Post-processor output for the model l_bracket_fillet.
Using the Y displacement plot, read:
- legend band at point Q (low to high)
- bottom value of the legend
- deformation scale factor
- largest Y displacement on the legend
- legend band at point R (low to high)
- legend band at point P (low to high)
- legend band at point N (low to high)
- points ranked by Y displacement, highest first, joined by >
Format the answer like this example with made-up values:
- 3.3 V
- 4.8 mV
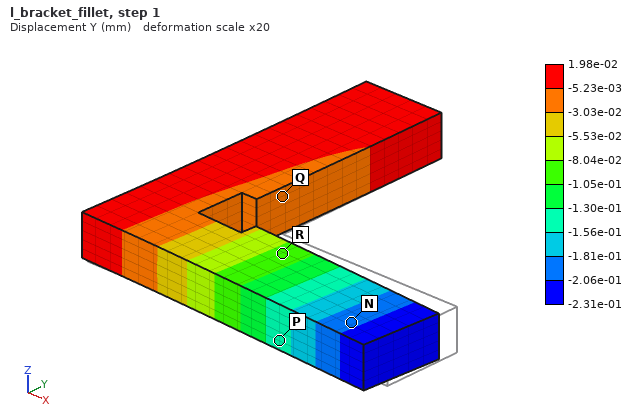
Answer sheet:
- -3.03e-02 to -5.23e-03 mm
- -2.31e-01 mm
- 20
- 1.98e-02 mm
- -1.05e-01 to -8.04e-02 mm
- -1.56e-01 to -1.30e-01 mm
- -2.06e-01 to -1.81e-01 mm
- Q > R > P > N
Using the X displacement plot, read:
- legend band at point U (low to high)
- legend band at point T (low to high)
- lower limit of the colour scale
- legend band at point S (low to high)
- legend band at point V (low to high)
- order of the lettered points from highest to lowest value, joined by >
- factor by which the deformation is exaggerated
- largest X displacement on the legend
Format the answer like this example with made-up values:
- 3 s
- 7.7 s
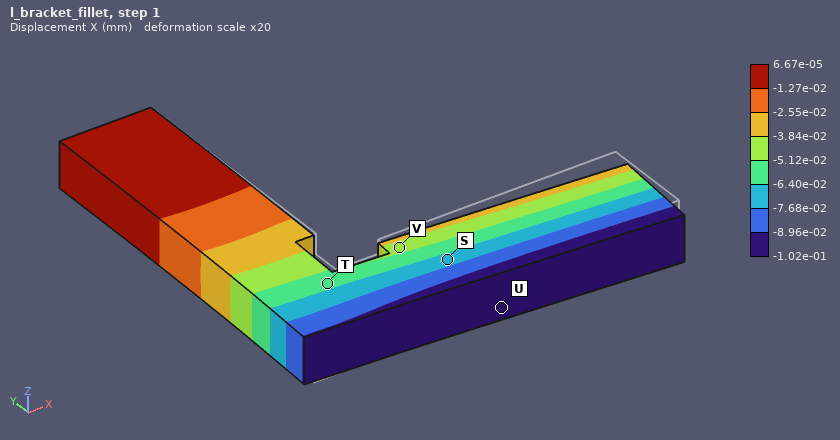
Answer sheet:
- -1.02e-01 to -8.96e-02 mm
- -6.40e-02 to -5.12e-02 mm
- -1.02e-01 mm
- -7.68e-02 to -6.40e-02 mm
- -5.12e-02 to -3.84e-02 mm
- V > T > S > U
- 20
- 6.67e-05 mm
